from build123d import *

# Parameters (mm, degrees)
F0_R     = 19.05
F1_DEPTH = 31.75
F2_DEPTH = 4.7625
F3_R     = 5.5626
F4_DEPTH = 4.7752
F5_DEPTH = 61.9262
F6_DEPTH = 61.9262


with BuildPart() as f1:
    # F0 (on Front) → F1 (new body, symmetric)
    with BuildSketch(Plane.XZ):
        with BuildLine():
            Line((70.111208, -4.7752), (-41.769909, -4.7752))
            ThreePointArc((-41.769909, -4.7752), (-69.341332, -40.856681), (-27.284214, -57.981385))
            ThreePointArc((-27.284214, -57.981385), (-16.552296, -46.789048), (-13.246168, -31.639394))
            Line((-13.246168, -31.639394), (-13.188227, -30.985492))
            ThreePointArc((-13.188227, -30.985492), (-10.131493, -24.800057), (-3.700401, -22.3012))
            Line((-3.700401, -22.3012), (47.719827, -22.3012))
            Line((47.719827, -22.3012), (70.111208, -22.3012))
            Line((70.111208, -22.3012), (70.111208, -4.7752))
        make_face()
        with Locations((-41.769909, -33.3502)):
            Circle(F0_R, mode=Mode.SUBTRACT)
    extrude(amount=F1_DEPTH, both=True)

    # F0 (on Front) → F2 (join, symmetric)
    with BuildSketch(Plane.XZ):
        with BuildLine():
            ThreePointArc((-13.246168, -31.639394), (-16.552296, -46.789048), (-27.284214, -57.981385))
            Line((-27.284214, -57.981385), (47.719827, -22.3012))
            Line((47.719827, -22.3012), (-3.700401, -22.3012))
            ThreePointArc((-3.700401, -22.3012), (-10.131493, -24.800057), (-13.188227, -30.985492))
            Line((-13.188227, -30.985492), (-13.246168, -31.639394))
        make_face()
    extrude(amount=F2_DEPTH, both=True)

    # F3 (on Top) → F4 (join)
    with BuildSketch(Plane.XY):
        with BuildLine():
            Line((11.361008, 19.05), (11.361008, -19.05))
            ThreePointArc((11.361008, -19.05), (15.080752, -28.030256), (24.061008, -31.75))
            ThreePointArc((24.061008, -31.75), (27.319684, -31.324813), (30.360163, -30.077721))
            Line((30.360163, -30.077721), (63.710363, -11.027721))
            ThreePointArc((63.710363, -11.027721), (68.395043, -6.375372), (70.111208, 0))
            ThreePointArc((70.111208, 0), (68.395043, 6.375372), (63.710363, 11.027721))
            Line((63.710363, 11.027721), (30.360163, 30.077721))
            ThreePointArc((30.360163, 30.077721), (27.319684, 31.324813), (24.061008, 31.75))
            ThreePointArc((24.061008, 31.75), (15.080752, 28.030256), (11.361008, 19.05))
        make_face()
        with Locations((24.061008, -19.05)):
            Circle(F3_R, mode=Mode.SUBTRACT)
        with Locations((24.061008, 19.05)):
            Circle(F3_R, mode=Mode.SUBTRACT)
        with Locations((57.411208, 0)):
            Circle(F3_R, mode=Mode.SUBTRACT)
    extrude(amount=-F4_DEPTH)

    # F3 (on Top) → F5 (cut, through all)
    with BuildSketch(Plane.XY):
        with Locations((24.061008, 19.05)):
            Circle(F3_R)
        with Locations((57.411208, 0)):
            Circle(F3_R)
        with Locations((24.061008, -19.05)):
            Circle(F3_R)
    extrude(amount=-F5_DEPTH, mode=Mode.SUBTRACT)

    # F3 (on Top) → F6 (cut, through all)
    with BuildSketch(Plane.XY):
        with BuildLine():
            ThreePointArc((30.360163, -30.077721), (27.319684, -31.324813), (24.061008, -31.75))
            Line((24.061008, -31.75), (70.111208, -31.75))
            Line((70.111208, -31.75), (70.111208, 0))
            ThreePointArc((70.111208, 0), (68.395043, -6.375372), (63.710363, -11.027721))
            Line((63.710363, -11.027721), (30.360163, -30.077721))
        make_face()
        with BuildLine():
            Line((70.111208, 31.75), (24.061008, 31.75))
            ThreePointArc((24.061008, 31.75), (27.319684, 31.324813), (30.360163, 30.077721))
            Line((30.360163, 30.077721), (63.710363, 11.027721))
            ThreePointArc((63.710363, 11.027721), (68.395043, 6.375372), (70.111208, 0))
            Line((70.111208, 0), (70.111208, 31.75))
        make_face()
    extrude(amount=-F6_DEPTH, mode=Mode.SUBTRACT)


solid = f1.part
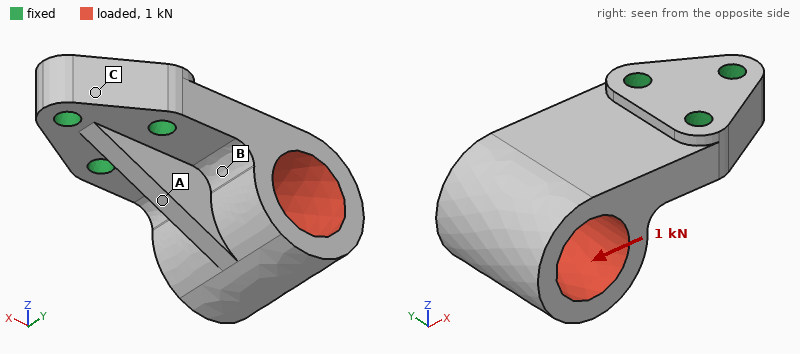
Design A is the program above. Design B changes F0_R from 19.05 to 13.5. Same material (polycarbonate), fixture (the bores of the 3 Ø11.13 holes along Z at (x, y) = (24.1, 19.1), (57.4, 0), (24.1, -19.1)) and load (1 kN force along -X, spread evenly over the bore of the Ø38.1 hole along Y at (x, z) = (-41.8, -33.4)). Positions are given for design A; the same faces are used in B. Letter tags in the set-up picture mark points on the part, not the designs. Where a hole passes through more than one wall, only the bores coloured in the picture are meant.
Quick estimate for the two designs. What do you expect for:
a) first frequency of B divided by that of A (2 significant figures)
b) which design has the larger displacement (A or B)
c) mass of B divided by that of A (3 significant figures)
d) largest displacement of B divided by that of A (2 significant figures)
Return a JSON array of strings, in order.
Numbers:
["0.90", "A", "1.19", "0.89"]
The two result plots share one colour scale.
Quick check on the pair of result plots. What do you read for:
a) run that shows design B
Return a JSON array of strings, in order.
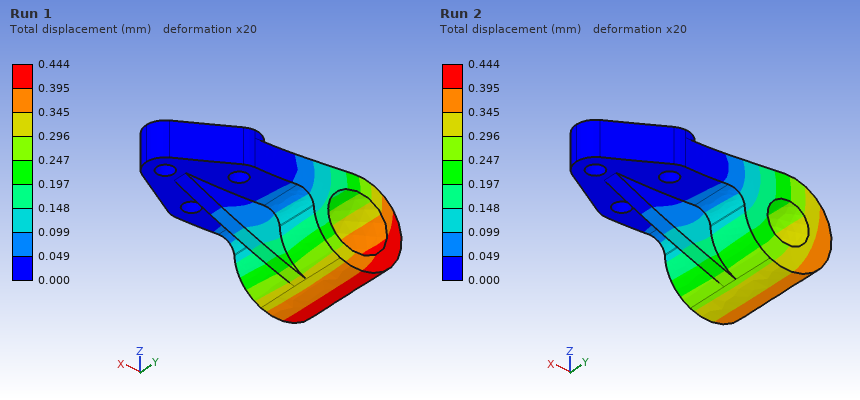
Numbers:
["Run 2"]
